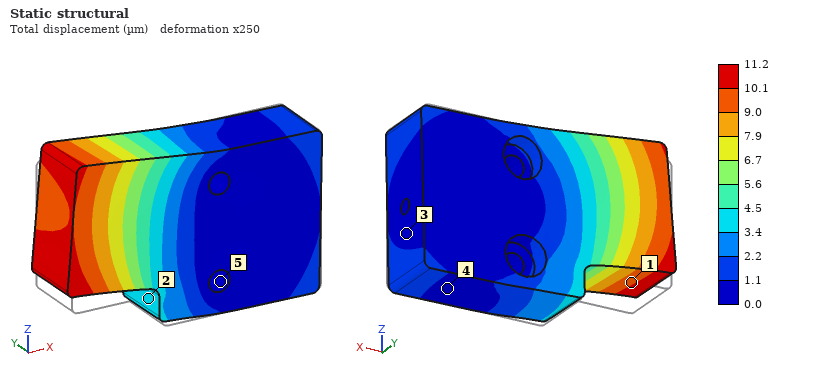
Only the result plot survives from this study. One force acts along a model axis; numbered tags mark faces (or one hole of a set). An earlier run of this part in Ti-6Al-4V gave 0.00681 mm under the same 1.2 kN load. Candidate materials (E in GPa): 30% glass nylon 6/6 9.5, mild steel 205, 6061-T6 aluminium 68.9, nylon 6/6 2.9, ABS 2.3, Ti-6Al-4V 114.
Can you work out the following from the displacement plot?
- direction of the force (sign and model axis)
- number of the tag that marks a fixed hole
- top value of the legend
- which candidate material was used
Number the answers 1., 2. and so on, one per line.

1. +Z
2. 5
3. 11.2 µm
4. 6061-T6 aluminium
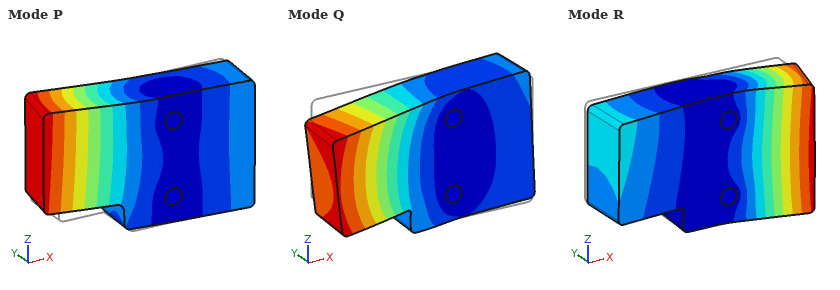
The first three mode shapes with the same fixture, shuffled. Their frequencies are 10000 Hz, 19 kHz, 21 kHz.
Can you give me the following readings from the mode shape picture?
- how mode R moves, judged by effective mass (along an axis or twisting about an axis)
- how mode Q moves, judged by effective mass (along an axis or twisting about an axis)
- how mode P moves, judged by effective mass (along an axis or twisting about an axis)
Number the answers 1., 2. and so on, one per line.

1. along Y
2. along Z
3. along Y
